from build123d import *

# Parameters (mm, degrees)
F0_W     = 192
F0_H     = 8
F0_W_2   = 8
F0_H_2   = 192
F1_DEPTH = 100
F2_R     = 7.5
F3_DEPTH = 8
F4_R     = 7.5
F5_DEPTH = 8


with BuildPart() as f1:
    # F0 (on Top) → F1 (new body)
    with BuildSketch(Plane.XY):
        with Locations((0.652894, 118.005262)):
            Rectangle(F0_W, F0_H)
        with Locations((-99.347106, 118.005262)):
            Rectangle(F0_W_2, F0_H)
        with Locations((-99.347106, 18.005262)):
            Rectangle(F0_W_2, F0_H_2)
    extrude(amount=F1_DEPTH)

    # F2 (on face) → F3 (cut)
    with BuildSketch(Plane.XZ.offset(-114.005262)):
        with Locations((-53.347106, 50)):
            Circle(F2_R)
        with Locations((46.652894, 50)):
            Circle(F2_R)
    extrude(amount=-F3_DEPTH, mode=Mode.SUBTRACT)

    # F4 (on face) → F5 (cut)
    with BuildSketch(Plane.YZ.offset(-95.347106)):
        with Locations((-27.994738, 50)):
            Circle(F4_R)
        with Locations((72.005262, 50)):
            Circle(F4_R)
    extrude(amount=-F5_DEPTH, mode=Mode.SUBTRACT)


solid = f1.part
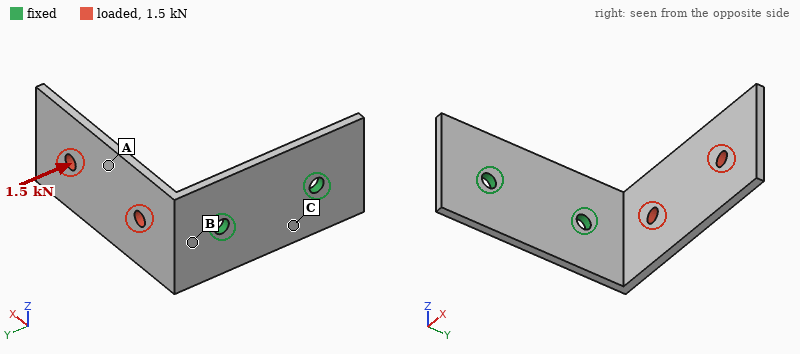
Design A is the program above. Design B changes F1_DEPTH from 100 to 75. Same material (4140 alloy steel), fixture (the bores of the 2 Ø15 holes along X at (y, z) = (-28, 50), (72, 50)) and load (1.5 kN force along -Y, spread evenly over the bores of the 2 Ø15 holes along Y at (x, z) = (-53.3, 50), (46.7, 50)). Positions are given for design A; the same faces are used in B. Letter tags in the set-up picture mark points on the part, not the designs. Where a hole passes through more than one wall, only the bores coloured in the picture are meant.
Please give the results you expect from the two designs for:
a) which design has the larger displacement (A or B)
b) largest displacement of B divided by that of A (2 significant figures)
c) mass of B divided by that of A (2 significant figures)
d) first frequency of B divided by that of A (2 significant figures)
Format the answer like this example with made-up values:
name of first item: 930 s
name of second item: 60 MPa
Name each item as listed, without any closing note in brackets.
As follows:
which design has the larger displacement: B
largest displacement of B divided by that of A: 1.3
mass of B divided by that of A: 0.75
first frequency of B divided by that of A: 1.0
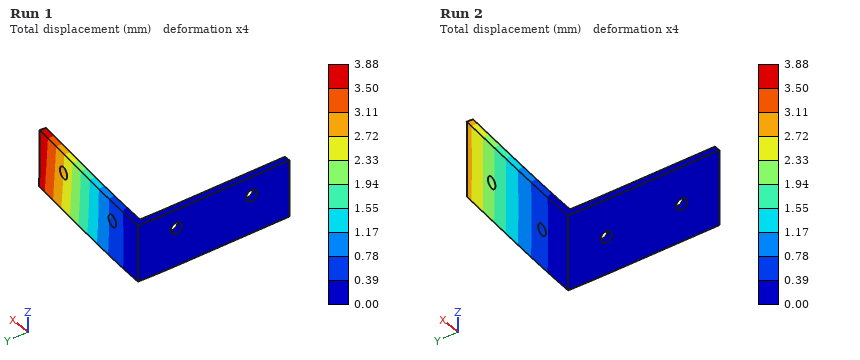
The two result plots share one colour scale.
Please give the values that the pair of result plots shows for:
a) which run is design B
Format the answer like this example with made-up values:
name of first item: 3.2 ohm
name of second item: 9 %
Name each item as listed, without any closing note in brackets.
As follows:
which run is design B: Run 1
